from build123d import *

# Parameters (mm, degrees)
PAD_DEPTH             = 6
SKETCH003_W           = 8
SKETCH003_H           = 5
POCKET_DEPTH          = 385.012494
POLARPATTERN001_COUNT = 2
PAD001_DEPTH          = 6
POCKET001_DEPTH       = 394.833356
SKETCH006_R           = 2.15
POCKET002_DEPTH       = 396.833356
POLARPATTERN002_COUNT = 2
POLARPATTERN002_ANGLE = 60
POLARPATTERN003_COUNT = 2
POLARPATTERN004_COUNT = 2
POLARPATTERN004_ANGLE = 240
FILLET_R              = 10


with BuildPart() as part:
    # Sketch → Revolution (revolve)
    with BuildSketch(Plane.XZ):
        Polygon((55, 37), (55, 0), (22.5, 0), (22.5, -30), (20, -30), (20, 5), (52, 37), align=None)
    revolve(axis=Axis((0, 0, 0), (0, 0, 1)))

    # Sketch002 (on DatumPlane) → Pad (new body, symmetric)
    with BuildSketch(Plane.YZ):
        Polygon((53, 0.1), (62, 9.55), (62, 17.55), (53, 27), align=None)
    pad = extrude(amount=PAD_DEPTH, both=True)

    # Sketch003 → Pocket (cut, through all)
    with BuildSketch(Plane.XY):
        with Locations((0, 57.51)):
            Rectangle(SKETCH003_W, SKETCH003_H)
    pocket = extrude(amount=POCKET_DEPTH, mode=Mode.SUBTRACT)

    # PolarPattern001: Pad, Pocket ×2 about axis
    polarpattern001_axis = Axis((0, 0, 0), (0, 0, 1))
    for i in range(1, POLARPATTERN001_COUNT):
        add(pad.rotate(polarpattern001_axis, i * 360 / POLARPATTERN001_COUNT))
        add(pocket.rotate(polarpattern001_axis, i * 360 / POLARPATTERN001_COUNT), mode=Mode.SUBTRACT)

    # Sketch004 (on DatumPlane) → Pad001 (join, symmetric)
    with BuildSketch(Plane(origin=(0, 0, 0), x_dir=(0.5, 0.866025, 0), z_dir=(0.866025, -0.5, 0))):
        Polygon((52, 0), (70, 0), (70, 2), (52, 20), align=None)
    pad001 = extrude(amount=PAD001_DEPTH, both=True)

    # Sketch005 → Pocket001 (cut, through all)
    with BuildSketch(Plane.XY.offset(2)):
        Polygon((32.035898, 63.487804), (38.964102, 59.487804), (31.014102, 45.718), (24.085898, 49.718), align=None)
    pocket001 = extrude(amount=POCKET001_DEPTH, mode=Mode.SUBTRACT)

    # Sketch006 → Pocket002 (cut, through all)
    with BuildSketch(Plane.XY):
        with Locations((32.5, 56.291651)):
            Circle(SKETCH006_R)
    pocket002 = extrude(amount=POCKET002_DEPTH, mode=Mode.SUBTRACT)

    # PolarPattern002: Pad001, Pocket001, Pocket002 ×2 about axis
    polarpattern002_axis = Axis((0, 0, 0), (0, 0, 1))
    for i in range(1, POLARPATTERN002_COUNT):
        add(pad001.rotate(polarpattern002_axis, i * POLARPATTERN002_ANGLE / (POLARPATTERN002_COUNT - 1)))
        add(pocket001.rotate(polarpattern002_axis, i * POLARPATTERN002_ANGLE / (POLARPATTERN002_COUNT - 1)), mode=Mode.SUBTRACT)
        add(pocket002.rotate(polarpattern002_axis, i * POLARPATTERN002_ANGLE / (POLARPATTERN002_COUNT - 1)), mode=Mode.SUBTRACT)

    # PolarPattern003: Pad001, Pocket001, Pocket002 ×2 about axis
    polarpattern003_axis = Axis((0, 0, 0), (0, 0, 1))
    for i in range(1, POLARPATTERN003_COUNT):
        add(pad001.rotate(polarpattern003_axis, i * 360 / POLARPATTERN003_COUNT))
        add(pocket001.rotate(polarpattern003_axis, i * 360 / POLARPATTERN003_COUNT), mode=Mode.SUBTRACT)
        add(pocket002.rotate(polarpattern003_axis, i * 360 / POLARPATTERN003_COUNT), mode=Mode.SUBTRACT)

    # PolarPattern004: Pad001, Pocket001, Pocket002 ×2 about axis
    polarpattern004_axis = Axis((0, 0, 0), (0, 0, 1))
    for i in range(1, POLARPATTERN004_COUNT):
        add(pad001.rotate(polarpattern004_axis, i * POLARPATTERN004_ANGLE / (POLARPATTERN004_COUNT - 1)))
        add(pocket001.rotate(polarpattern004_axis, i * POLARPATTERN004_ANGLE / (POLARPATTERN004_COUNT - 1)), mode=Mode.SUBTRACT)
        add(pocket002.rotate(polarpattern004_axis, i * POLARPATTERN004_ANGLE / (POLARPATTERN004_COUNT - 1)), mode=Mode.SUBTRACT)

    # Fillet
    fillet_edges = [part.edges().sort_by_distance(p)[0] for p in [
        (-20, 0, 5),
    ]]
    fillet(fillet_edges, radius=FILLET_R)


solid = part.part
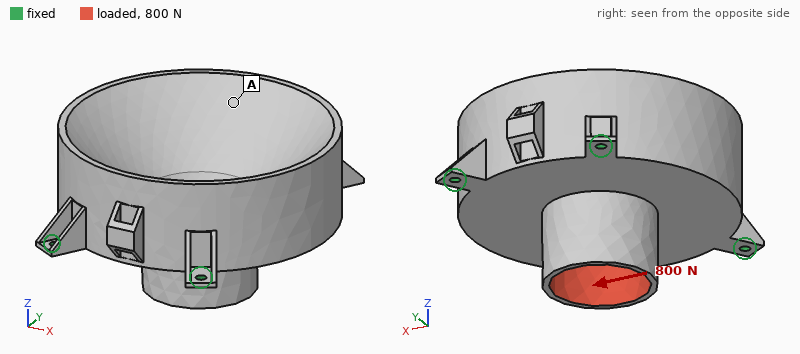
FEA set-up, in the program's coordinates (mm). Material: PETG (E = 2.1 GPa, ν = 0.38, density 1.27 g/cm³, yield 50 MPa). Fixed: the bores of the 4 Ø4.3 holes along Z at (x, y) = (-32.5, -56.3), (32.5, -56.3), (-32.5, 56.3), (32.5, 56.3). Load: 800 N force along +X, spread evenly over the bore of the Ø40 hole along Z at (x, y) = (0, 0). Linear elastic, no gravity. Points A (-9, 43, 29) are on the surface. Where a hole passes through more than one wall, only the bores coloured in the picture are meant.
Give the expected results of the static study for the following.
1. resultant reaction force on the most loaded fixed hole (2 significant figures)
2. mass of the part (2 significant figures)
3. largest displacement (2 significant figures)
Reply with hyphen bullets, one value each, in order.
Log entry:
- 230 N
- 280 g
- 0.47 mm
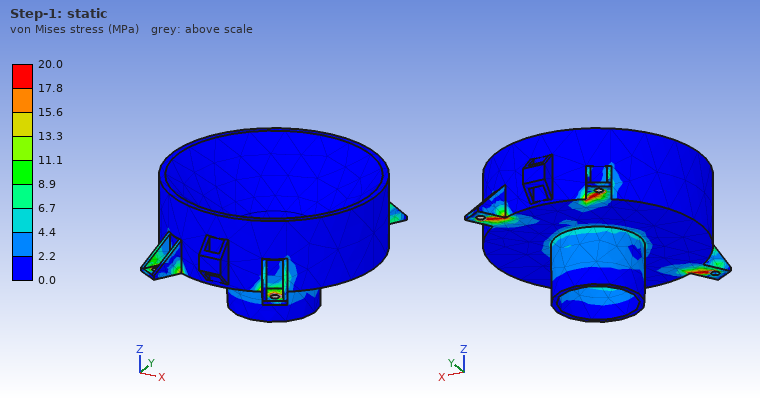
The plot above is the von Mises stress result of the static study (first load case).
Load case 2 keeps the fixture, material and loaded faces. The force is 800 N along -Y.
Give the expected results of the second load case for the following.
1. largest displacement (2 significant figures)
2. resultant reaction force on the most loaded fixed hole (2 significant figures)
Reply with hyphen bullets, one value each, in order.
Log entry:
- 0.34 mm
- 220 N
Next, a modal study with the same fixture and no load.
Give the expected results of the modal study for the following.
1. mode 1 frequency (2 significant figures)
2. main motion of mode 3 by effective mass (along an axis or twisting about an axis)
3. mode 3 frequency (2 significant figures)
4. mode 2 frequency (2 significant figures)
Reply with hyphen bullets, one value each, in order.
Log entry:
- 580 Hz
- along X
- 850 Hz
- 600 Hz
